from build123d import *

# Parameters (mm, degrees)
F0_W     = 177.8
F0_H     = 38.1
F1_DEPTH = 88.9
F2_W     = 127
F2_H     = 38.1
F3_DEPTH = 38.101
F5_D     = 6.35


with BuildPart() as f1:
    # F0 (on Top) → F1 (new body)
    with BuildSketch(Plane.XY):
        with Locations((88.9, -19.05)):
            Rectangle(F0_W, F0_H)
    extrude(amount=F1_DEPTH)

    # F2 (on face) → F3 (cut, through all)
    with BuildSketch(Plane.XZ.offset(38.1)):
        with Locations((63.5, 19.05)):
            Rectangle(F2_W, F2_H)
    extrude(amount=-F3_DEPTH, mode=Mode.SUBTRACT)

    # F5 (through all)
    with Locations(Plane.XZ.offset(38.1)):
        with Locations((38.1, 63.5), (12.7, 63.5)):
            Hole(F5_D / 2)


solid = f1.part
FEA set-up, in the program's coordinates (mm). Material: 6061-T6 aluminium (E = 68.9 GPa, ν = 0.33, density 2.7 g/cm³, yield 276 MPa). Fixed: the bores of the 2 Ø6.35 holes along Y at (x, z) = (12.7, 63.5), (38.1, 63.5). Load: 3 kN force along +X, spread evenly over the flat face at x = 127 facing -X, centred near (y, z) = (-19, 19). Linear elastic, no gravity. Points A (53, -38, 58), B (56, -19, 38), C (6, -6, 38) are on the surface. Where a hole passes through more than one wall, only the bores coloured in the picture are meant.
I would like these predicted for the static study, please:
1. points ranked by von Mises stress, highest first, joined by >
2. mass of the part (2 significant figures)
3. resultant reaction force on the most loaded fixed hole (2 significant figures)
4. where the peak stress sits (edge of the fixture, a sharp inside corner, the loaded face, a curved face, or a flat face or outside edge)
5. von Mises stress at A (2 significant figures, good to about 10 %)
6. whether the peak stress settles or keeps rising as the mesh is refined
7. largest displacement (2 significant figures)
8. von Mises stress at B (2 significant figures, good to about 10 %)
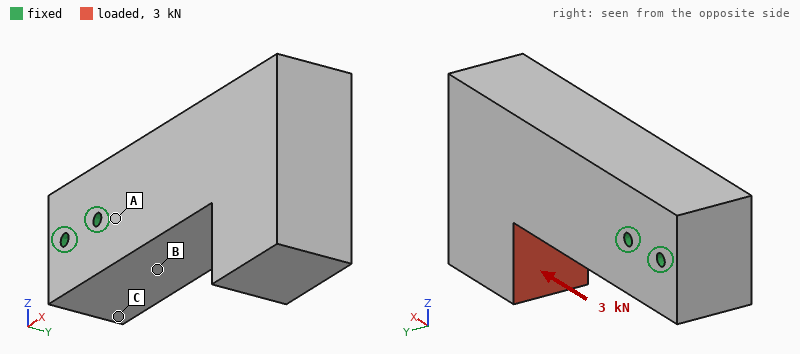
B > A > C
1.1 kg
4.7 kN
edge of the fixture
3.6 MPa
keeps rising
81 µm
9.6 MPa
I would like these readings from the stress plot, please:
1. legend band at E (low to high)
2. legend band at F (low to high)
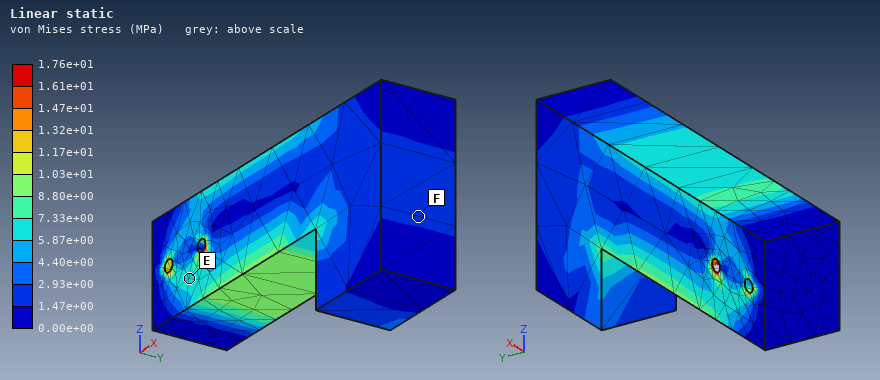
5.87e+00 to 7.33e+00 MPa
1.47e+00 to 2.93e+00 MPa
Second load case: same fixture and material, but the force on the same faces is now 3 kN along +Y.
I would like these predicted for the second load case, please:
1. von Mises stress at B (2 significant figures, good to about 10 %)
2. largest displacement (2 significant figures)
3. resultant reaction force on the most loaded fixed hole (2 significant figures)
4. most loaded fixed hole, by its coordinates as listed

14 MPa
0.18 mm
5.1 kN
(38.1, 63.5)
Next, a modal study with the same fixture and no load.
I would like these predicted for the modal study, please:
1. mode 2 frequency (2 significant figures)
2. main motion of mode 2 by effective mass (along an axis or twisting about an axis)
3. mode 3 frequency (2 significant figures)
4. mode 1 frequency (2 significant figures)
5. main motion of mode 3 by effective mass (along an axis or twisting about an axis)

1100 Hz
along Z
2700 Hz
1000 Hz
twisting about X
